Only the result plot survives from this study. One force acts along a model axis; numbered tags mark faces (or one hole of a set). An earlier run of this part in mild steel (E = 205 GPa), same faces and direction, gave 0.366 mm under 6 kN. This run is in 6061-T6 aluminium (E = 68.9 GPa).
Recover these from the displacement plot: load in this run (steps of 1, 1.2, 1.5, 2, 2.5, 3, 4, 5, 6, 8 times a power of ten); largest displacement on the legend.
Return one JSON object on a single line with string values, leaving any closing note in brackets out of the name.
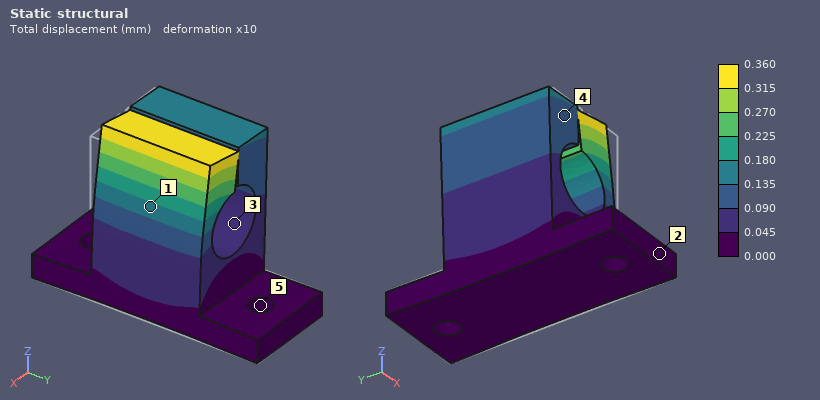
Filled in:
{"load in this run": "2 kN", "largest displacement on the legend": "0.360 mm"}
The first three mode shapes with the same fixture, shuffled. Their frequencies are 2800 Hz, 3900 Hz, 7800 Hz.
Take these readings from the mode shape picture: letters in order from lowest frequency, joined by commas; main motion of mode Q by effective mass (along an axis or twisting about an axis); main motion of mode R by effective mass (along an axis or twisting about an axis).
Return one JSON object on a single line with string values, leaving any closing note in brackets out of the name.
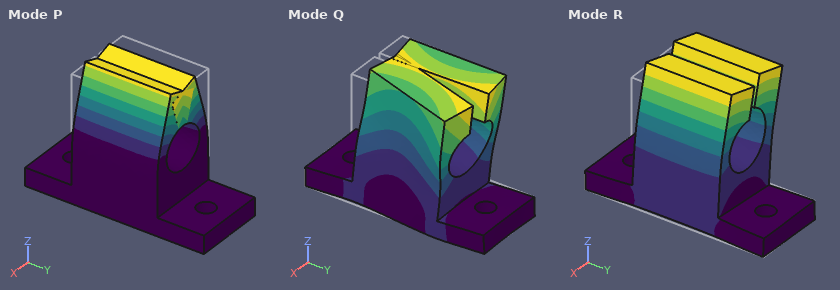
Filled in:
{"letters in order from lowest frequency, joined by commas": "R, P, Q", "main motion of mode Q by effective mass": "along Y", "main motion of mode R by effective mass": "along X"}
